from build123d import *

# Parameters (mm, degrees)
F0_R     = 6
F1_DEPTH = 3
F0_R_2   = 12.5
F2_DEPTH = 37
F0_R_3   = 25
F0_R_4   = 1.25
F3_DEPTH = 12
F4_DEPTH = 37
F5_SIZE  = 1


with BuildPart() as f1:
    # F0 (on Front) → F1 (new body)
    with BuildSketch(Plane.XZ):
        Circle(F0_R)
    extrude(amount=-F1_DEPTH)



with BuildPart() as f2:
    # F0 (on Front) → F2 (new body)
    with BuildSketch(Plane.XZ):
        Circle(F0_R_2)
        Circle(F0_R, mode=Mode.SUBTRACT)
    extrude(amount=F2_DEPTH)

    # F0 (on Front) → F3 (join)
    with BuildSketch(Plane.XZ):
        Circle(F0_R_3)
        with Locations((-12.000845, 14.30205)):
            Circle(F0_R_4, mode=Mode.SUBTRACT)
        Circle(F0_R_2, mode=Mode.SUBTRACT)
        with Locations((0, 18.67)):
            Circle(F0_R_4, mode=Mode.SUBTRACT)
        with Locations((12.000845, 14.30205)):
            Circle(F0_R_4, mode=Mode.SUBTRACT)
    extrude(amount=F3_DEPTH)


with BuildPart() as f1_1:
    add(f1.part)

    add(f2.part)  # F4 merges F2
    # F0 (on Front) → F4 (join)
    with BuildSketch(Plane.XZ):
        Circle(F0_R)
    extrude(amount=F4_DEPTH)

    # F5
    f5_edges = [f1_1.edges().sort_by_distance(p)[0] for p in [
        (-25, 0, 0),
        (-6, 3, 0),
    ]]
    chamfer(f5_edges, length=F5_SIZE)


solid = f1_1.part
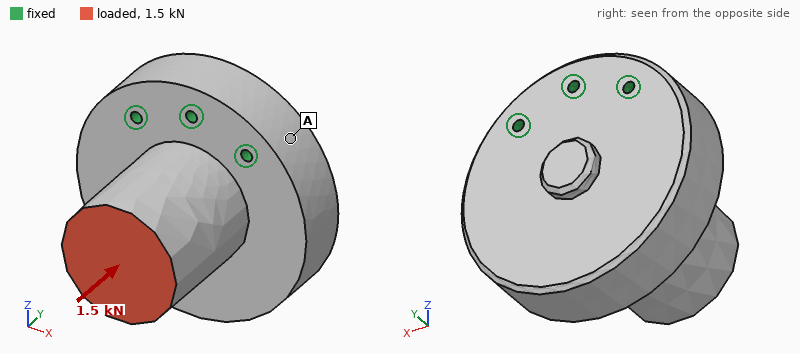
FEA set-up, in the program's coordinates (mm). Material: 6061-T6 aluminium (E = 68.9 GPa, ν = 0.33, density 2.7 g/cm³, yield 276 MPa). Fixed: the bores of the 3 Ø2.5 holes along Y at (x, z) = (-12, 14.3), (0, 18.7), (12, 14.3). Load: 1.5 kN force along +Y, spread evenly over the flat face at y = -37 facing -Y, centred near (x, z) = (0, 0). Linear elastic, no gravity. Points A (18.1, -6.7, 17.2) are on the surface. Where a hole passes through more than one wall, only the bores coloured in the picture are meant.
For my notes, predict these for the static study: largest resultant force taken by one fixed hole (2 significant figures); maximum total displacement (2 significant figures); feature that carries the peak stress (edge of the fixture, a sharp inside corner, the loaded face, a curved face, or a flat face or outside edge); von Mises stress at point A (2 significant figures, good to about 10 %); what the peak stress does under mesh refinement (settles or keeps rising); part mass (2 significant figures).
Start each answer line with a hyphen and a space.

- 720 N
- 23 µm
- edge of the fixture
- 7.0 MPa
- keeps rising
- 97 g
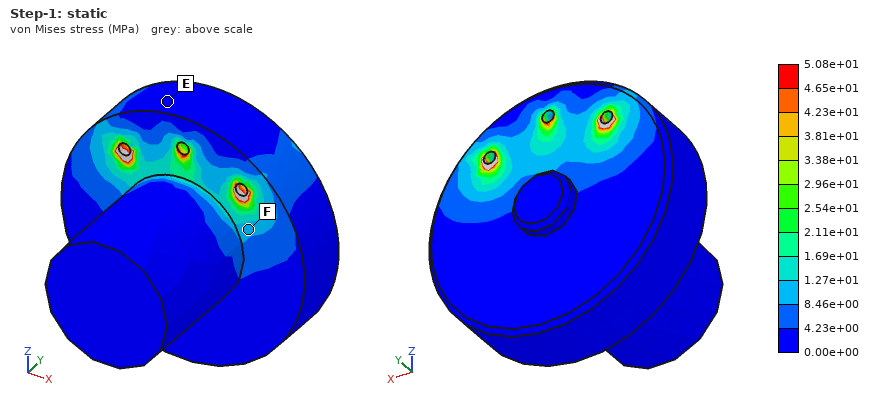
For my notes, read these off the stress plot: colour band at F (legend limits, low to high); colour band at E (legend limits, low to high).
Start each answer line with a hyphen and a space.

- 8.46e+00 to 1.27e+01 MPa
- 0.00e+00 to 4.23e+00 MPa
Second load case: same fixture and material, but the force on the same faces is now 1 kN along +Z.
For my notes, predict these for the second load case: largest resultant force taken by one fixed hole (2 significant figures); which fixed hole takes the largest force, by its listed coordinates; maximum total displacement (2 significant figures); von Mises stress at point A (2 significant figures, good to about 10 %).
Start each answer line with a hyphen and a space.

- 770 N
- (0, 18.7)
- 45 µm
- 12 MPa
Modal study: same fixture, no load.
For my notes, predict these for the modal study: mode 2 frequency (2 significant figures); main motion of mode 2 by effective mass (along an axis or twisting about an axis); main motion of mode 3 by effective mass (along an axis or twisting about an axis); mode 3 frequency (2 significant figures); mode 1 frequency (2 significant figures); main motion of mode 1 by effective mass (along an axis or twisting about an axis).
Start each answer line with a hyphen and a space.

- 8700 Hz
- along X
- along X
- 12 kHz
- 4500 Hz
- along Y
